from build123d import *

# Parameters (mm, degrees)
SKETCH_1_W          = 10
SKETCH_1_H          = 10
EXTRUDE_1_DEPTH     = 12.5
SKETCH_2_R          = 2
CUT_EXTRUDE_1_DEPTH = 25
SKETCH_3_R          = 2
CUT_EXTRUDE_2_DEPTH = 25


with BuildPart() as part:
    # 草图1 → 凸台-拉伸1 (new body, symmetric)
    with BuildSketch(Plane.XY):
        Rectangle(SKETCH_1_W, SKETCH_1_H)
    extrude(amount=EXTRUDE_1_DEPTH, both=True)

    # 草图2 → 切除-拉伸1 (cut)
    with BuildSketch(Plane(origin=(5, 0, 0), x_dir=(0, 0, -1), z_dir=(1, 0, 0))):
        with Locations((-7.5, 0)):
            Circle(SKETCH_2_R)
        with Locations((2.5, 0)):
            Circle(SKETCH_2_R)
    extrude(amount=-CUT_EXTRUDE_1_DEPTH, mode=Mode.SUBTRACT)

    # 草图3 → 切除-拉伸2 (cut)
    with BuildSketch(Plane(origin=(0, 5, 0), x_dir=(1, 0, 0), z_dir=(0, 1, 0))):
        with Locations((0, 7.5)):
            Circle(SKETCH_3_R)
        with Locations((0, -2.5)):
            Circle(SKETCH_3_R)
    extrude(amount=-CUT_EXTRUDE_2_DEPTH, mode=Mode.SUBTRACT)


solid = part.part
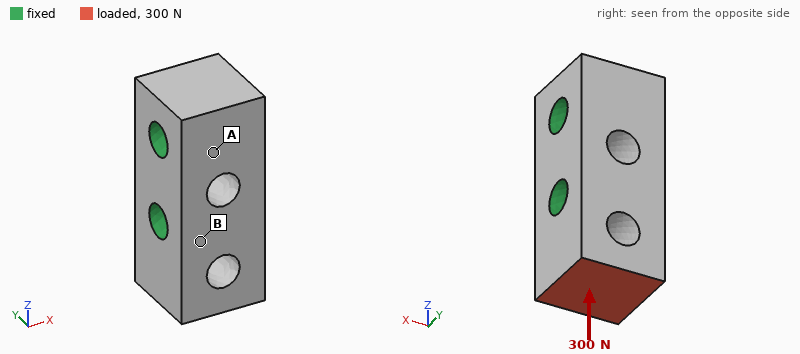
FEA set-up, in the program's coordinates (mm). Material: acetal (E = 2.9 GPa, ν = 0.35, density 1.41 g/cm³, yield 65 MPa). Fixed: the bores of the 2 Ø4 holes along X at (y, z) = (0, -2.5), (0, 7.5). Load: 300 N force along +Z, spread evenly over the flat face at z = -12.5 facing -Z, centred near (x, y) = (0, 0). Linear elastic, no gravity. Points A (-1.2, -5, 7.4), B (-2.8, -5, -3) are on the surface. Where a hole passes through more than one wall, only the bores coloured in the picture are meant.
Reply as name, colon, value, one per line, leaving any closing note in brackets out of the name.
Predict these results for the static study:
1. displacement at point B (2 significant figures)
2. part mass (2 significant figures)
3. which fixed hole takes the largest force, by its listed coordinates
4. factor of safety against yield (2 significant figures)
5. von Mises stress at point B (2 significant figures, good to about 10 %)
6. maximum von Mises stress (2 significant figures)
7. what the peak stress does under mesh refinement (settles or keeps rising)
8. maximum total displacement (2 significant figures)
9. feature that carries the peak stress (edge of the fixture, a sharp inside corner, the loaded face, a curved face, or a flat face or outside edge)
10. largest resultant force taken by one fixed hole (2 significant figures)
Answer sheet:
displacement at point B: 3.3 µm
part mass: 2.8 g
which fixed hole takes the largest force, by its listed coordinates: (0, -2.5)
factor of safety against yield: 5.2
von Mises stress at point B: 2.1 MPa
maximum von Mises stress: 12 MPa
what the peak stress does under mesh refinement: settles
maximum total displacement: 18 µm
feature that carries the peak stress: a curved face
largest resultant force taken by one fixed hole: 280 N
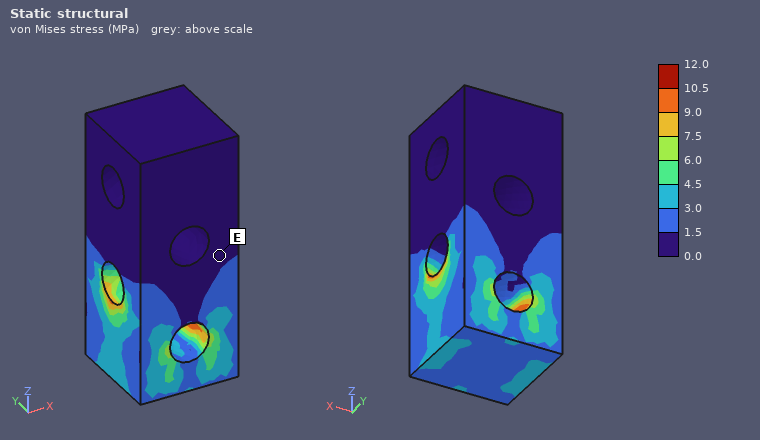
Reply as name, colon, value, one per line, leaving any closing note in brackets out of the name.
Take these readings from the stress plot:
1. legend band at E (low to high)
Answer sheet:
legend band at E: 0.0 to 1.5 MPa
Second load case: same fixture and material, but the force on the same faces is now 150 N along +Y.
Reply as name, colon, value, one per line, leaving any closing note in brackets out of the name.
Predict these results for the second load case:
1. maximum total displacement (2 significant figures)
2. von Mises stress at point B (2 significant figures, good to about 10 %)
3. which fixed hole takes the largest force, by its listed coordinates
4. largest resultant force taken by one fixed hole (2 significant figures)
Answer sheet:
maximum total displacement: 67 µm
von Mises stress at point B: 6.6 MPa
which fixed hole takes the largest force, by its listed coordinates: (0, -2.5)
largest resultant force taken by one fixed hole: 190 N
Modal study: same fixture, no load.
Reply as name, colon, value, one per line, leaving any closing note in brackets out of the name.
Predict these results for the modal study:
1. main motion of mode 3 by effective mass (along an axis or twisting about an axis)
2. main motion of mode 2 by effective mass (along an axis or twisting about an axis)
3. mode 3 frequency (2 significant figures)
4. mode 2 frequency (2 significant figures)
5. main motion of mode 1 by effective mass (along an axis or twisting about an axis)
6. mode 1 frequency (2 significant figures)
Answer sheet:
main motion of mode 3 by effective mass: twisting about Z
main motion of mode 2 by effective mass: along X
mode 3 frequency: 19 kHz
mode 2 frequency: 14 kHz
main motion of mode 1 by effective mass: along Y
mode 1 frequency: 13 kHz
